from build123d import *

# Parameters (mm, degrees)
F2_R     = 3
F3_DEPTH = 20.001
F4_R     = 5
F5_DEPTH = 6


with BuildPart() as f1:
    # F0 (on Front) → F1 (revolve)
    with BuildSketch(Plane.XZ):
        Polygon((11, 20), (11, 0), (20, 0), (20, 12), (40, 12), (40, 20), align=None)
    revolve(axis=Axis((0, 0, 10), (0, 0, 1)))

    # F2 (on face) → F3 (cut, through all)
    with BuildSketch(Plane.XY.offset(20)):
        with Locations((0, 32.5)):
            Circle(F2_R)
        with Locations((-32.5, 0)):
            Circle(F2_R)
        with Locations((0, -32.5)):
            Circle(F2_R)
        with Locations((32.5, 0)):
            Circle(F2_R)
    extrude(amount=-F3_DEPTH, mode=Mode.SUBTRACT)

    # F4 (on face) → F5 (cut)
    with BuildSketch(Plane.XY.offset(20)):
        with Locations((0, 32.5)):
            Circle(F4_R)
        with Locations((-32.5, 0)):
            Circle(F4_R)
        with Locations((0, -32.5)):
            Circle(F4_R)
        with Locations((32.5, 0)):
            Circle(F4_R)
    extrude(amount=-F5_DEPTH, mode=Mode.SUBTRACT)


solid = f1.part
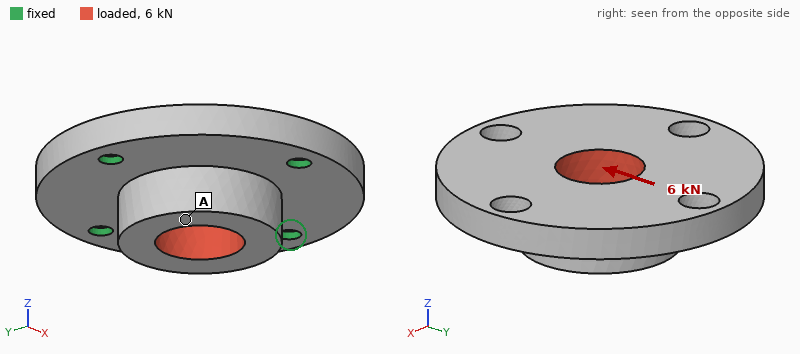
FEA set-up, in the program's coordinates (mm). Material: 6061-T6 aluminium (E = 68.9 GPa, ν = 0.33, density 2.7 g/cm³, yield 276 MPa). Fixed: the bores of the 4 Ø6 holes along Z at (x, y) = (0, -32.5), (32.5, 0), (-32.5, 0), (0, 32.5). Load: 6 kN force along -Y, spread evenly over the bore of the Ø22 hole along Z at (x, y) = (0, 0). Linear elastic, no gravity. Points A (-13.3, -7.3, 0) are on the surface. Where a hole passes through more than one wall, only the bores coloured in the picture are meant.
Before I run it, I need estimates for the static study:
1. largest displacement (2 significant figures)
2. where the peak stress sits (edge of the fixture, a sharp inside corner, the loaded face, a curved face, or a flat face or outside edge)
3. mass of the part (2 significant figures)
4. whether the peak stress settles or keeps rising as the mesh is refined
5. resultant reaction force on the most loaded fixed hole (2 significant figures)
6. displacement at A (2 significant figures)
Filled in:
14 µm
edge of the fixture
120 g
keeps rising
1.5 kN
12 µm
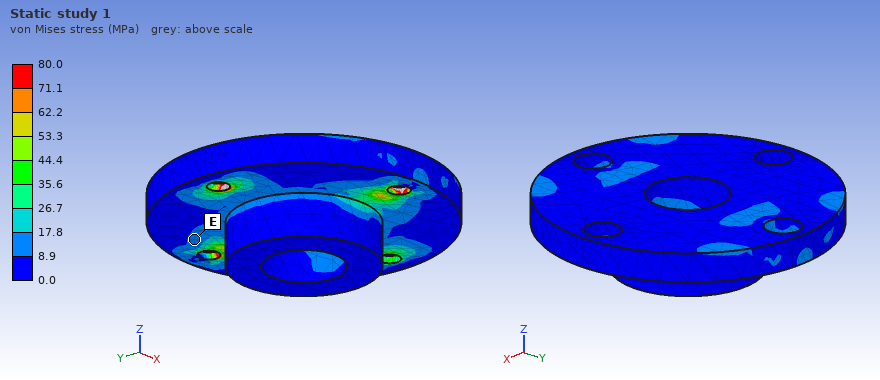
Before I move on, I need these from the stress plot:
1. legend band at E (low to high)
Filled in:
8.9 to 17.8 MPa
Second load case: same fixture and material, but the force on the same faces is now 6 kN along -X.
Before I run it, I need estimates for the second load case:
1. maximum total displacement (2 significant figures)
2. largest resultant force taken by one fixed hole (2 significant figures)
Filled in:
14 µm
1.5 kN
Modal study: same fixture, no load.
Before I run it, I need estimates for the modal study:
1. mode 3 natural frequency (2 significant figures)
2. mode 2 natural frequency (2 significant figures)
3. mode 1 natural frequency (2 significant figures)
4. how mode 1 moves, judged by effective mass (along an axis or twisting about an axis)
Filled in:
10000 Hz
9900 Hz
9000 Hz
along Z
